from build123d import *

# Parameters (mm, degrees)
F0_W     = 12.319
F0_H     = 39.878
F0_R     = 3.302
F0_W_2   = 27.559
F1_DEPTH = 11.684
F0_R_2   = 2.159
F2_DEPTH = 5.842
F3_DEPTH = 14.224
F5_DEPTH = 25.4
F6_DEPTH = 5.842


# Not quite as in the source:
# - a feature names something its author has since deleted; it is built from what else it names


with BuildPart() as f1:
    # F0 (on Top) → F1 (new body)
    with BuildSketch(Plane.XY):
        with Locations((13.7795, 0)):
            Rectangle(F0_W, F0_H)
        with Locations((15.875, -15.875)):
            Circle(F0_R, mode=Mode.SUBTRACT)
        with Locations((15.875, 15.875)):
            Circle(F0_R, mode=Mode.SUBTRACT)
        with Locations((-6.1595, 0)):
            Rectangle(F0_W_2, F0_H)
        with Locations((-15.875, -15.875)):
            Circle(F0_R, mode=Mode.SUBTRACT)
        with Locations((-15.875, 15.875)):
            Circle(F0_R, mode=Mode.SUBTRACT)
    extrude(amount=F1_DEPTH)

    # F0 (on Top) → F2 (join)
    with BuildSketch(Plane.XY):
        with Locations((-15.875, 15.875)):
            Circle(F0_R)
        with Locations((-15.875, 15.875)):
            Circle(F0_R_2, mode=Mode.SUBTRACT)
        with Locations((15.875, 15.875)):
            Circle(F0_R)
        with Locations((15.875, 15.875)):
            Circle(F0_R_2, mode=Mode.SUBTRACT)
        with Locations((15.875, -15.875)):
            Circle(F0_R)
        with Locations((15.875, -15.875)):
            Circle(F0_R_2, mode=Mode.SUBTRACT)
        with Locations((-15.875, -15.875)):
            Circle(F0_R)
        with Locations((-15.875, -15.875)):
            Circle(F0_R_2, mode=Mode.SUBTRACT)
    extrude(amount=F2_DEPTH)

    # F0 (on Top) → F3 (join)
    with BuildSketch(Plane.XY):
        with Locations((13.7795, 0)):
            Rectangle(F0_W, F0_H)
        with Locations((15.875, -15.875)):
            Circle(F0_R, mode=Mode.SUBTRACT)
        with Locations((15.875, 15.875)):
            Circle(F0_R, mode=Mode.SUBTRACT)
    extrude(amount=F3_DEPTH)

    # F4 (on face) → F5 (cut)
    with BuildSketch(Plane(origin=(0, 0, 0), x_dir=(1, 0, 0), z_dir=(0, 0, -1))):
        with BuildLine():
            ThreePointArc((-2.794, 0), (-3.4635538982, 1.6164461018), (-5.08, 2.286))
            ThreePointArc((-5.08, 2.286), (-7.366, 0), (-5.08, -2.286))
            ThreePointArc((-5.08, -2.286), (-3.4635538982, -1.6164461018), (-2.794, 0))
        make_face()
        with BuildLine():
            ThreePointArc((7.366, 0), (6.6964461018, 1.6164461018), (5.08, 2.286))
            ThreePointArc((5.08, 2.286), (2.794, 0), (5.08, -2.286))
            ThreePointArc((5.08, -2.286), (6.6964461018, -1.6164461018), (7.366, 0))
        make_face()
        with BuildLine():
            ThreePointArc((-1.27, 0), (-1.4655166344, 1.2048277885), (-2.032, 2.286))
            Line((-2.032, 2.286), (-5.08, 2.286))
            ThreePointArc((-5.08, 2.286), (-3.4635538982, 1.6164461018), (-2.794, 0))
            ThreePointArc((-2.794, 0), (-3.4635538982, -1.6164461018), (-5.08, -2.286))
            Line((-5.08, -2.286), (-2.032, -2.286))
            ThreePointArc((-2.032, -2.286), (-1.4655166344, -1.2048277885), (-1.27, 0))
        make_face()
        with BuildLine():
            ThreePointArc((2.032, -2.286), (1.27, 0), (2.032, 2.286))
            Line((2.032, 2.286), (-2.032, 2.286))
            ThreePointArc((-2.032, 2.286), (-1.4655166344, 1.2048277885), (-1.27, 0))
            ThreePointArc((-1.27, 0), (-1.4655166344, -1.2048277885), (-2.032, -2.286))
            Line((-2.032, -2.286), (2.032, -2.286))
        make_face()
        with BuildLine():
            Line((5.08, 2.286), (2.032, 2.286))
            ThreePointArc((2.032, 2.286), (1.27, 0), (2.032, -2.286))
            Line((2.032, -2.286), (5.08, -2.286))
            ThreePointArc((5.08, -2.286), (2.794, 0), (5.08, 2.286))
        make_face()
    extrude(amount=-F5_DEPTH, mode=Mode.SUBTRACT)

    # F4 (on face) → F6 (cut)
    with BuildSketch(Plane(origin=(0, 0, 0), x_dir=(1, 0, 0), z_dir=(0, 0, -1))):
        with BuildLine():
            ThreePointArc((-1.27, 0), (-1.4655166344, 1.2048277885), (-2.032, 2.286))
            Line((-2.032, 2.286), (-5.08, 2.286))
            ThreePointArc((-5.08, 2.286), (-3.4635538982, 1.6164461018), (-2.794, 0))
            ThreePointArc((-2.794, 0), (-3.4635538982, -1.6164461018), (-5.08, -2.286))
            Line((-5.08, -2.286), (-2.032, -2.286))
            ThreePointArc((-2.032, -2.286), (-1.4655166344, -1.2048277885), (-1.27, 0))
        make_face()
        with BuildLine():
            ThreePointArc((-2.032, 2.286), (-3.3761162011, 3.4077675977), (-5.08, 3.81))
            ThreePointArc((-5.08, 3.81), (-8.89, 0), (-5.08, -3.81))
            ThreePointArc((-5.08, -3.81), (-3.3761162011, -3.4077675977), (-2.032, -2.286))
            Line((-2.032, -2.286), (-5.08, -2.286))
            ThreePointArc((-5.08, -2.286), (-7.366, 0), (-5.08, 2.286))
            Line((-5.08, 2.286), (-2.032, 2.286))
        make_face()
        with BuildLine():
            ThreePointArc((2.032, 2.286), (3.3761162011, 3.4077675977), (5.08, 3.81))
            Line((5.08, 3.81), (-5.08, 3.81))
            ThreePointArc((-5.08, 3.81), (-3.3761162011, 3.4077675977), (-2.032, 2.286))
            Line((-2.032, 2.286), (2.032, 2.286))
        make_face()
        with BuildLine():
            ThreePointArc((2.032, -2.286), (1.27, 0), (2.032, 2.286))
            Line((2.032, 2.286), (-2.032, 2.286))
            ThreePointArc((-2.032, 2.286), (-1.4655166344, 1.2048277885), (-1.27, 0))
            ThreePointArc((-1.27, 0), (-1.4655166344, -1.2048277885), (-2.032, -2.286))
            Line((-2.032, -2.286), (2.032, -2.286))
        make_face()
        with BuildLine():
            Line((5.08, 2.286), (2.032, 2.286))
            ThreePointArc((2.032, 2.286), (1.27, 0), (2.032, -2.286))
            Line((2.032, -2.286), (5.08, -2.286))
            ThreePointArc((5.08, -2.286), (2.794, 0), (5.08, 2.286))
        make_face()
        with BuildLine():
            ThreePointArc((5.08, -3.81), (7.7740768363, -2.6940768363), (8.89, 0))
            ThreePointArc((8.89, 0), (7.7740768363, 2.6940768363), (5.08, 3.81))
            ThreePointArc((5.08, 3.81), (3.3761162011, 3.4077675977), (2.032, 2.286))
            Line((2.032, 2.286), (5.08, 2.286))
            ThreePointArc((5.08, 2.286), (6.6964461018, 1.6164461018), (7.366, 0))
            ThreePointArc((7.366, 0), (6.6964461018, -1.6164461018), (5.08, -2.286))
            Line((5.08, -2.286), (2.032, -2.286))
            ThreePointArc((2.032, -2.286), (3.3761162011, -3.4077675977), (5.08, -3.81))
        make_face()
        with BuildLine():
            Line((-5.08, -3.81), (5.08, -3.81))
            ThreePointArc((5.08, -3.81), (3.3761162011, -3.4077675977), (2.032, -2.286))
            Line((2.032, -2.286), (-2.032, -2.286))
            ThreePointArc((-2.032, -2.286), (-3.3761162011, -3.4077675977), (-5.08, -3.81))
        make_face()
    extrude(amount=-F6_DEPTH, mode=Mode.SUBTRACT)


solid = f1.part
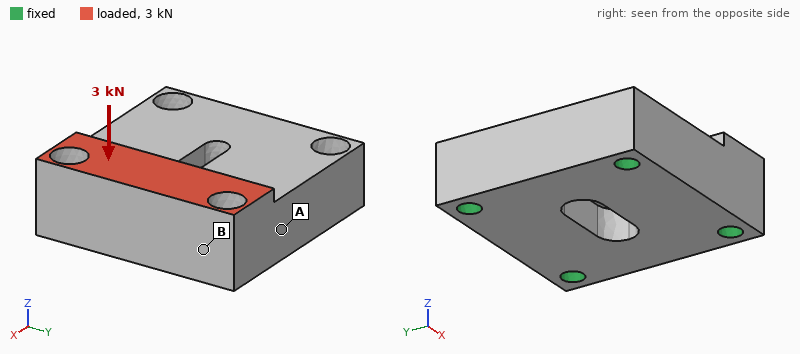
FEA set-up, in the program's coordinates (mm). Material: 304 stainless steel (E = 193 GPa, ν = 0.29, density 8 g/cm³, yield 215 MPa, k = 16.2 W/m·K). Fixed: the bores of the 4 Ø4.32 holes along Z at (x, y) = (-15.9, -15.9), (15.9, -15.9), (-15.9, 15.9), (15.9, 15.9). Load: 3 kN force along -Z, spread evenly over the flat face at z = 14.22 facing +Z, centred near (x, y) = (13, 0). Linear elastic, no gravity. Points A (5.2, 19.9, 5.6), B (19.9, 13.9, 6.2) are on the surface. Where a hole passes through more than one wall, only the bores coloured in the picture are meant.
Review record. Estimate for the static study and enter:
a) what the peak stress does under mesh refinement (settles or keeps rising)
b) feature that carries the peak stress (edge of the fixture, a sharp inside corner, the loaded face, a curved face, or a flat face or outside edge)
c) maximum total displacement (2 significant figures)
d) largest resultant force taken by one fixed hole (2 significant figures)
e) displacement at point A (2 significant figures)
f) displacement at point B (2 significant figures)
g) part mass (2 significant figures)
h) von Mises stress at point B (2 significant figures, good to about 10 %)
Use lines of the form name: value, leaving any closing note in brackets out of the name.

what the peak stress does under mesh refinement: keeps rising
feature that carries the peak stress: edge of the fixture
maximum total displacement: 2.3 µm
largest resultant force taken by one fixed hole: 1.5 kN
displacement at point A: 0.55 µm
displacement at point B: 0.72 µm
part mass: 140 g
von Mises stress at point B: 22 MPa
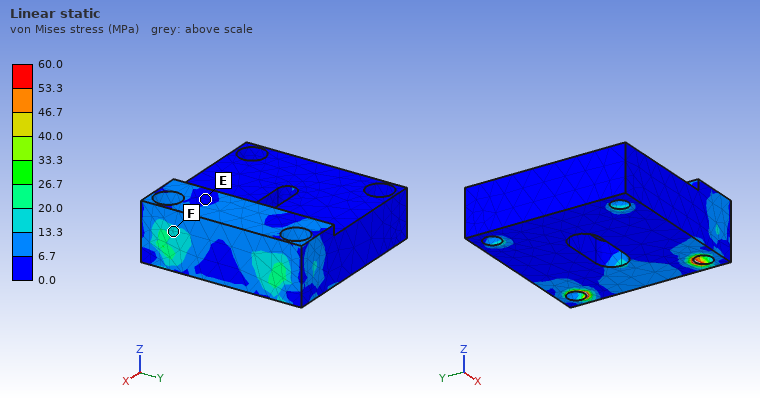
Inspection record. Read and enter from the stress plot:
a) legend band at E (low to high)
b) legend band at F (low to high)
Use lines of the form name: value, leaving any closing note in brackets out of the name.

legend band at E: 0.0 to 6.7 MPa
legend band at F: 13.3 to 20.0 MPa
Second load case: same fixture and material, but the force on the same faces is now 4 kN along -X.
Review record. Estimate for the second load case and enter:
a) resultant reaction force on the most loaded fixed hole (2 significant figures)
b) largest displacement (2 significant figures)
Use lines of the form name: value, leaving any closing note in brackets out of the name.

resultant reaction force on the most loaded fixed hole: 1.4 kN
largest displacement: 5.2 µm
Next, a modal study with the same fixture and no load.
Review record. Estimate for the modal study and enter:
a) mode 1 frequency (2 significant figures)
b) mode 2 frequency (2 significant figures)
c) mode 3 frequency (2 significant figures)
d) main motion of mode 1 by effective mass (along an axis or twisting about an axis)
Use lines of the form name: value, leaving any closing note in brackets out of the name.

mode 1 frequency: 22 kHz
mode 2 frequency: 31 kHz
mode 3 frequency: 31 kHz
main motion of mode 1 by effective mass: along Z
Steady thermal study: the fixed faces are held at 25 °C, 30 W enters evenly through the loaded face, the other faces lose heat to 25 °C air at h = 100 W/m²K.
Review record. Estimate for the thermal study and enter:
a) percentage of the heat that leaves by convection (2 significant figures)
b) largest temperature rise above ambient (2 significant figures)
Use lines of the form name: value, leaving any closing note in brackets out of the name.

percentage of the heat that leaves by convection: 31 %
largest temperature rise above ambient: 65 K
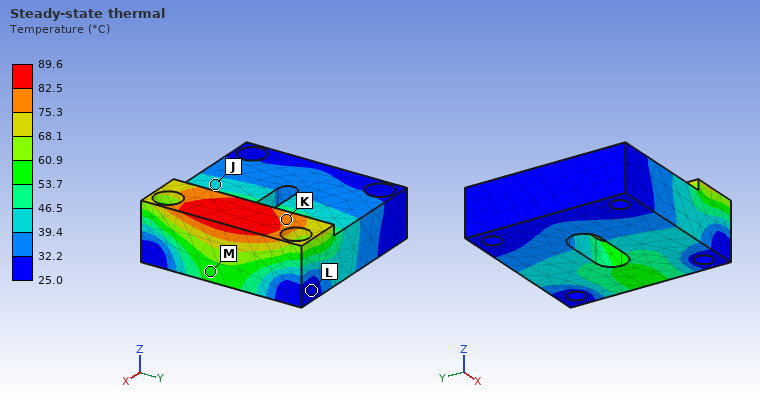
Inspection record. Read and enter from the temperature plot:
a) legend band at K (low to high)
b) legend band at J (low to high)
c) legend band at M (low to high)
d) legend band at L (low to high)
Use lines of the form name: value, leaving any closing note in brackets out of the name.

legend band at K: 75.3 to 82.5 °C
legend band at J: 39.4 to 46.5 °C
legend band at M: 53.7 to 60.9 °C
legend band at L: 25.0 to 32.2 °C
